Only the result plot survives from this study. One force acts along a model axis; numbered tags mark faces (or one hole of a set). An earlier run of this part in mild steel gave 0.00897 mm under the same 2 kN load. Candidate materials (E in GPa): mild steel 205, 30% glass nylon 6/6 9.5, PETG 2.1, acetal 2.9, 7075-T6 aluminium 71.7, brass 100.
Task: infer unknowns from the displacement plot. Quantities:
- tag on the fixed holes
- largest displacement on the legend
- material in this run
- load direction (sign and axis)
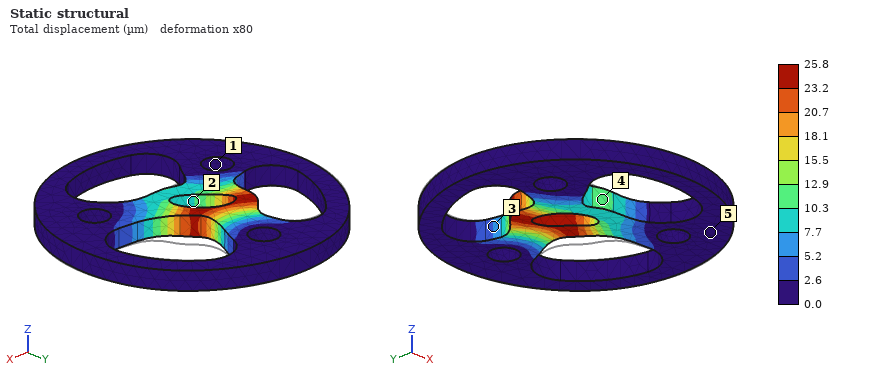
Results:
1
25.8 µm
7075-T6 aluminium
-X
